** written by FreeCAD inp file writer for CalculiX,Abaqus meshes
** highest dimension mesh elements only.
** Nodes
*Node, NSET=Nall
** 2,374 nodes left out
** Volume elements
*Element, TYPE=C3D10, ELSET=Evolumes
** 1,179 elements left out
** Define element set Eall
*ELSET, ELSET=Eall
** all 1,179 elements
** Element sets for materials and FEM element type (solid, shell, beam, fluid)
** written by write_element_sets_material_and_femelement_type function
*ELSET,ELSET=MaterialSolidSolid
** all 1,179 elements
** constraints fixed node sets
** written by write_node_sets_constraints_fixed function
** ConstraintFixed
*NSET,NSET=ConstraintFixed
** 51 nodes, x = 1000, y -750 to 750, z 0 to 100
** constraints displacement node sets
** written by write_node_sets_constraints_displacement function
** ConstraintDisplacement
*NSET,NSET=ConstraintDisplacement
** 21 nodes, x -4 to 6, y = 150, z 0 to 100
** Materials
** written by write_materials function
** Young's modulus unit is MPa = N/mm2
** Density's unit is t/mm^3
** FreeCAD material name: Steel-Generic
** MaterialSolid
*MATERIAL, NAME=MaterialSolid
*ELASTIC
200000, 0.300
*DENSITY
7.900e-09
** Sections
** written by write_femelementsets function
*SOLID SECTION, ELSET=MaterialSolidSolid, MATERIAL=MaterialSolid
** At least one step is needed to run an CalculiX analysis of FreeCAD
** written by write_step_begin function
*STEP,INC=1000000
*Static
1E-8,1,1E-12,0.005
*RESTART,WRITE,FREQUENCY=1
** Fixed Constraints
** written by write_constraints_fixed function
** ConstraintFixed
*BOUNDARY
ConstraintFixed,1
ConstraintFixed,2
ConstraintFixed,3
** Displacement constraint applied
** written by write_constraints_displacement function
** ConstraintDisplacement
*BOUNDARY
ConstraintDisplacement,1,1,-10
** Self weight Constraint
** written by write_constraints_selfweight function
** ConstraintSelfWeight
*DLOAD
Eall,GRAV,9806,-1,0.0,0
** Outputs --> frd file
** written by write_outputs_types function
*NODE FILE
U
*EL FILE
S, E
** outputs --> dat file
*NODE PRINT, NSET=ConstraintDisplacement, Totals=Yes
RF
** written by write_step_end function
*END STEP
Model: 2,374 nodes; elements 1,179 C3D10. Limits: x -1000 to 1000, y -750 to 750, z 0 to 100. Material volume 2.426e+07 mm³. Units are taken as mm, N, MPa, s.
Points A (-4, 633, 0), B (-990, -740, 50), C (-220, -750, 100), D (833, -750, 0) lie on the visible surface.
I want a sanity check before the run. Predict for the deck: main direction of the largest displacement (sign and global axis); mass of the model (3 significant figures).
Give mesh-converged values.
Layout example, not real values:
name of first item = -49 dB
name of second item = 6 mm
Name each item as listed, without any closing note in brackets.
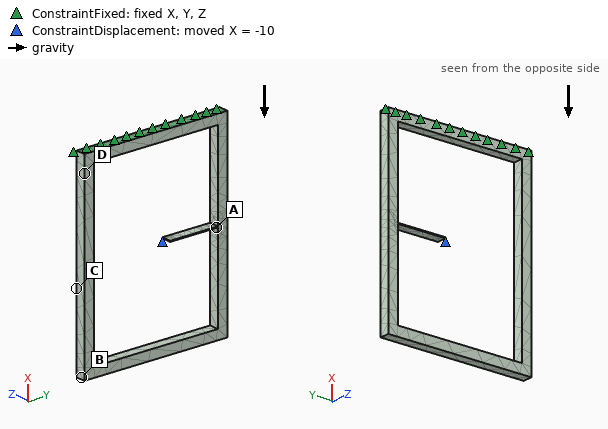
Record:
main direction of the largest displacement = -X
mass of the model = 192 kg
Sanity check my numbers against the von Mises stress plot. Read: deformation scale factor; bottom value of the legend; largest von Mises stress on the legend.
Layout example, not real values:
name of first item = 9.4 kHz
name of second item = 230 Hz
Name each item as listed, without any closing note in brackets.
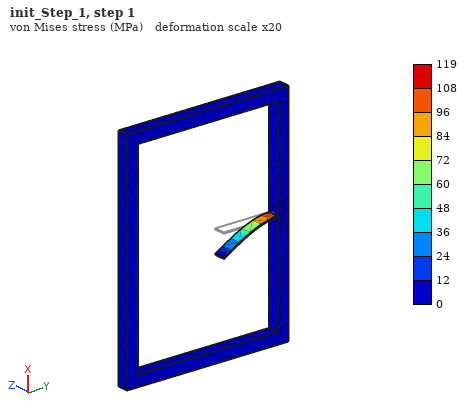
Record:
deformation scale factor = 20
bottom value of the legend = 0 MPa
largest von Mises stress on the legend = 119 MPa
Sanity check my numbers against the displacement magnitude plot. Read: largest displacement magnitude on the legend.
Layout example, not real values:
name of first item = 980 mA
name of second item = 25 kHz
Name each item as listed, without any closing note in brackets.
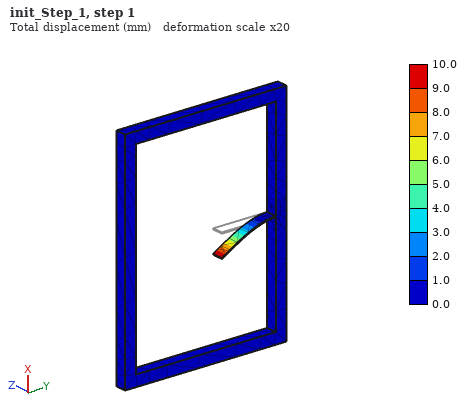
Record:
largest displacement magnitude on the legend = 10.0 mm
